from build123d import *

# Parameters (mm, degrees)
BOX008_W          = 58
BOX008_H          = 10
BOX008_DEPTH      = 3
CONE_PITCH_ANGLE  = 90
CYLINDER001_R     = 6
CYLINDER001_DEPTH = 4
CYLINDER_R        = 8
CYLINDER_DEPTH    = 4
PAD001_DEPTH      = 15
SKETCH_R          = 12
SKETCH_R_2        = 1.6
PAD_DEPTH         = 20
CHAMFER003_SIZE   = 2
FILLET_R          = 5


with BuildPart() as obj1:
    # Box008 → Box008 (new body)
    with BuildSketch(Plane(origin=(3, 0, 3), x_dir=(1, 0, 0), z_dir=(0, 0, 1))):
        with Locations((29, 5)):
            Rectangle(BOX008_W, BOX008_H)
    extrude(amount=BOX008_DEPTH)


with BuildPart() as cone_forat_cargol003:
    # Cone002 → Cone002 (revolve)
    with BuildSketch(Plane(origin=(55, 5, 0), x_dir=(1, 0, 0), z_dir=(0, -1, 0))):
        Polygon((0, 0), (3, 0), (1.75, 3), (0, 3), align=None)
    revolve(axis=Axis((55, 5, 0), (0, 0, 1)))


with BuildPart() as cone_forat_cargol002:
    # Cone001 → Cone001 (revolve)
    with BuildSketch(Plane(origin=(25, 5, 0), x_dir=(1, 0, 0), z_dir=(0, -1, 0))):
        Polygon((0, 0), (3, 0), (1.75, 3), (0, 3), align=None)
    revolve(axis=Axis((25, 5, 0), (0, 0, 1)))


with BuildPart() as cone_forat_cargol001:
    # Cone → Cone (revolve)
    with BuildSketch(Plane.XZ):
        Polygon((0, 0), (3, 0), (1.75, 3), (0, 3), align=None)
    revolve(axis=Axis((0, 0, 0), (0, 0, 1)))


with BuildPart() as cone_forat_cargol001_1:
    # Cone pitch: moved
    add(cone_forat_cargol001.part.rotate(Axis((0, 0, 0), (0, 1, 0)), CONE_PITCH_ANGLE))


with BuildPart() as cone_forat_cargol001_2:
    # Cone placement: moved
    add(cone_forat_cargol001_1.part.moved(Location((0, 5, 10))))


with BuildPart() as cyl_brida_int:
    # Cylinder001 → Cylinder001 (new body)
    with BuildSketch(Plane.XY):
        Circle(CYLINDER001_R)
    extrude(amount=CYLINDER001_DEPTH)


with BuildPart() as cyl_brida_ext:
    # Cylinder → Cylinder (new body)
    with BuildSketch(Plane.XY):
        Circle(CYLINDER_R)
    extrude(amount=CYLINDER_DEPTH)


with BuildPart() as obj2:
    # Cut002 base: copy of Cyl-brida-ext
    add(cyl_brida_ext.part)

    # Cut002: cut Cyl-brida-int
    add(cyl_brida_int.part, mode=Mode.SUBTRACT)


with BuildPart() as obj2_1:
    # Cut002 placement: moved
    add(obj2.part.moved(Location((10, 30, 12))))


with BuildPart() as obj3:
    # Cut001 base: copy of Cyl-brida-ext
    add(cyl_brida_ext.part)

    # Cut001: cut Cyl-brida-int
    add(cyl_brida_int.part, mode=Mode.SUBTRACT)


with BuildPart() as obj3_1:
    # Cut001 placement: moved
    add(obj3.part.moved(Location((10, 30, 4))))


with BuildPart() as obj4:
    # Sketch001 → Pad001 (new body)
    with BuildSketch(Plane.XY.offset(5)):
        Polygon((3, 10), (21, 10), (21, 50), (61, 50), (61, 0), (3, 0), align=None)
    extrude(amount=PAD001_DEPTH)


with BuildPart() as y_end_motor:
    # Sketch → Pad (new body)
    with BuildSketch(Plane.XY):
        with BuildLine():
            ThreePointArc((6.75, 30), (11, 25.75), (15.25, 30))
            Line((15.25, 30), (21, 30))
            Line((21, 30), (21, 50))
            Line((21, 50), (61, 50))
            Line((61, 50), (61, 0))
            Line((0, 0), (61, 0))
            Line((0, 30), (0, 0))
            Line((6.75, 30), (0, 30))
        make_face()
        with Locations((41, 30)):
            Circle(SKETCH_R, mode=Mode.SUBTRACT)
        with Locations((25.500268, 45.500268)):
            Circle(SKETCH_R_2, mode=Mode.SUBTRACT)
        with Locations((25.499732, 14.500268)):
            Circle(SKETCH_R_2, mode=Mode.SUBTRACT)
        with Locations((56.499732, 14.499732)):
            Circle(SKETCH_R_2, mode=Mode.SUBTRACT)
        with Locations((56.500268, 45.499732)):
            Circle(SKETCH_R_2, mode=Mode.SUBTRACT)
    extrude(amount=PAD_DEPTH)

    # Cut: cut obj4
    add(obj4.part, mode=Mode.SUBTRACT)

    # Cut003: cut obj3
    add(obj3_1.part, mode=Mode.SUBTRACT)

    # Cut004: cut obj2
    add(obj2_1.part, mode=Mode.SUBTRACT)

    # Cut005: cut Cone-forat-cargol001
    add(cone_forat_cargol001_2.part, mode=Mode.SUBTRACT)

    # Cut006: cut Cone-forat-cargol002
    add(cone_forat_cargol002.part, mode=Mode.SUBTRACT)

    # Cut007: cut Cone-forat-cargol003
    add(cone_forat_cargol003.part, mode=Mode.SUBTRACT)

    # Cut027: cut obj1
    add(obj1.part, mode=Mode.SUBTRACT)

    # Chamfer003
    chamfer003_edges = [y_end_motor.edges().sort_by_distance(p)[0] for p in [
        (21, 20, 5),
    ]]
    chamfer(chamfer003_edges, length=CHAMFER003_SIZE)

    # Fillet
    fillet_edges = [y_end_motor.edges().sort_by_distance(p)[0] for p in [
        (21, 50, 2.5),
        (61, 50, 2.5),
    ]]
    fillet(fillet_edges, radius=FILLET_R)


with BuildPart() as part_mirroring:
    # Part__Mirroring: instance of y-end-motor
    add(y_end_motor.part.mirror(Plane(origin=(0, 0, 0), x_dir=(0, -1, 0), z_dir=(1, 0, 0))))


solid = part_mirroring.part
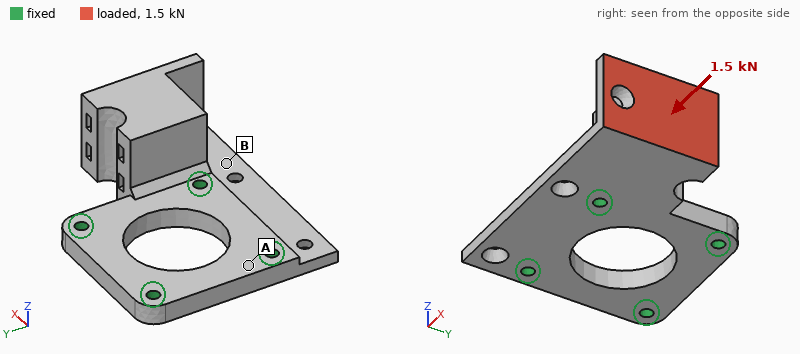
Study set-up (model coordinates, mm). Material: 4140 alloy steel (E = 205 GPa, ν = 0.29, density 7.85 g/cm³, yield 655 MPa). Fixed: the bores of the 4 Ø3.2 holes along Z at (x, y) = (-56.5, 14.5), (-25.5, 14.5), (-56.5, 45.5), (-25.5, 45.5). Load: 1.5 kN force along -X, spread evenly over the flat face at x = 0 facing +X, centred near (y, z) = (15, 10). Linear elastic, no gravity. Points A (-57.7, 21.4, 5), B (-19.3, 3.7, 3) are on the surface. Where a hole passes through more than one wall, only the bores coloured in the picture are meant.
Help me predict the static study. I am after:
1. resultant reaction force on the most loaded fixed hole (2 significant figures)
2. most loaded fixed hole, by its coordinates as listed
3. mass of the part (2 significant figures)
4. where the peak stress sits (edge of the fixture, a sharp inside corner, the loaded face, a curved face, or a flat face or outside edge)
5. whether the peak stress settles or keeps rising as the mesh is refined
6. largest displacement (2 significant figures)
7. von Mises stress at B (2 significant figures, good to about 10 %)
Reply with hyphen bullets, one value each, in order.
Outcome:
- 1.4 kN
- (-25.5, 14.5)
- 120 g
- edge of the fixture
- keeps rising
- 57 µm
- 26 MPa
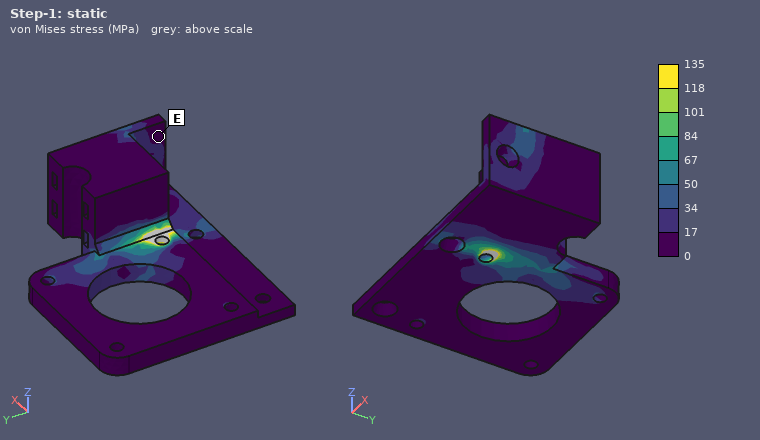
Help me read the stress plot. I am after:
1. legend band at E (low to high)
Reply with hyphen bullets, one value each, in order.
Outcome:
- 0 to 17 MPa
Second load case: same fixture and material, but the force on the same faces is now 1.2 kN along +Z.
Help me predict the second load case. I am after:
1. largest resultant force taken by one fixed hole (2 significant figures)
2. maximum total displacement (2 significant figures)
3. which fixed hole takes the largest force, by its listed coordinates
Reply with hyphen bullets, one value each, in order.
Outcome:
- 1.4 kN
- 0.13 mm
- (-25.5, 14.5)
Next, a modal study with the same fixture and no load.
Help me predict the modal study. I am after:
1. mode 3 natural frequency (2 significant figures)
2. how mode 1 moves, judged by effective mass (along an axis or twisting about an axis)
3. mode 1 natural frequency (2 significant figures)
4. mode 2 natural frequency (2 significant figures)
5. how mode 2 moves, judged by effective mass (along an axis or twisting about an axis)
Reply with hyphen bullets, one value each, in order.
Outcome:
- 9800 Hz
- along Z
- 2900 Hz
- 6200 Hz
- along Y
